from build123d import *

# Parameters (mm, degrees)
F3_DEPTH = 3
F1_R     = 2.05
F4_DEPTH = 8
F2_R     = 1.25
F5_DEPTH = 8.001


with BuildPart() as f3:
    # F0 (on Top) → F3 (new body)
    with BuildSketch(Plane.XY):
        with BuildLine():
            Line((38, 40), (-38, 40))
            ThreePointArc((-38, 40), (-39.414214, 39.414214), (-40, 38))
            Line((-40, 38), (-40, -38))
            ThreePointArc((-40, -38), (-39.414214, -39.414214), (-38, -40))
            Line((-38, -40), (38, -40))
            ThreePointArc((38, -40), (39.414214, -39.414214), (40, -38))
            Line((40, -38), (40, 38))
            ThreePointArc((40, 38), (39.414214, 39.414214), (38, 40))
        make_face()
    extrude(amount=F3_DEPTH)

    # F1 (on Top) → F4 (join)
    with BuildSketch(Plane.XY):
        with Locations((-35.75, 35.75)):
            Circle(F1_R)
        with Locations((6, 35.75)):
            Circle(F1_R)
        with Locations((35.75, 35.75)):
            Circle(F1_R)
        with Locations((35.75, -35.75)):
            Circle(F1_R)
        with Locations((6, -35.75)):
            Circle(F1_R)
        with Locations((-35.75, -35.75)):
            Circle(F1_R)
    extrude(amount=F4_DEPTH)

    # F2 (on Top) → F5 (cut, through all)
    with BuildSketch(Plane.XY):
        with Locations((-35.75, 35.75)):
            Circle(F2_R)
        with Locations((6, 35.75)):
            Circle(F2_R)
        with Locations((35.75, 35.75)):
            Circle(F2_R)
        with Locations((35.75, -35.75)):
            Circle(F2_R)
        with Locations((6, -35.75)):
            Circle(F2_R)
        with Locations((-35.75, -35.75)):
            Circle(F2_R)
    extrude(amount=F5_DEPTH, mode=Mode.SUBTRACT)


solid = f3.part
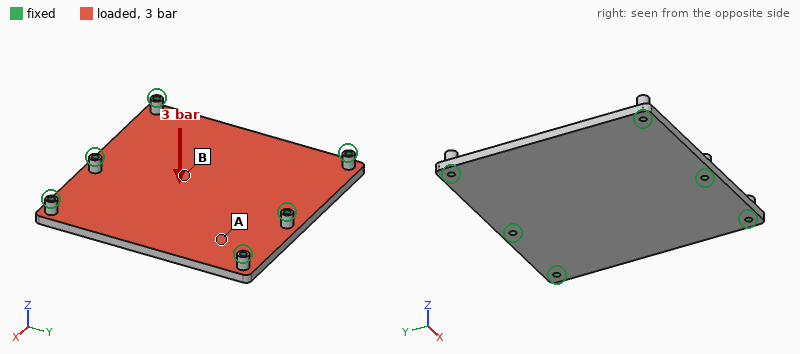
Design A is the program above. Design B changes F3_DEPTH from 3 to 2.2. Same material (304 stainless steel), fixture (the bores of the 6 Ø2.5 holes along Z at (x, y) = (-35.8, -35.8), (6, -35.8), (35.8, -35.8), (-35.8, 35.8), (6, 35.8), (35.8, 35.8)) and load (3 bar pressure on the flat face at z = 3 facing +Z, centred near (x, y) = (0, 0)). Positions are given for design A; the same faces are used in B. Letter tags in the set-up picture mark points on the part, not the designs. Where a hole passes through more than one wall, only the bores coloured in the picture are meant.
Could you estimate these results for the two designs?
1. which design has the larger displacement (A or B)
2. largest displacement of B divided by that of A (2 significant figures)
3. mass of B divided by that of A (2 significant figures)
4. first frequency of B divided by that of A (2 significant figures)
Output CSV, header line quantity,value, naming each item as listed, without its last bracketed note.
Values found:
quantity,value
which design has the larger displacement,B
largest displacement of B divided by that of A,2.4
mass of B divided by that of A,0.74
first frequency of B divided by that of A,0.75
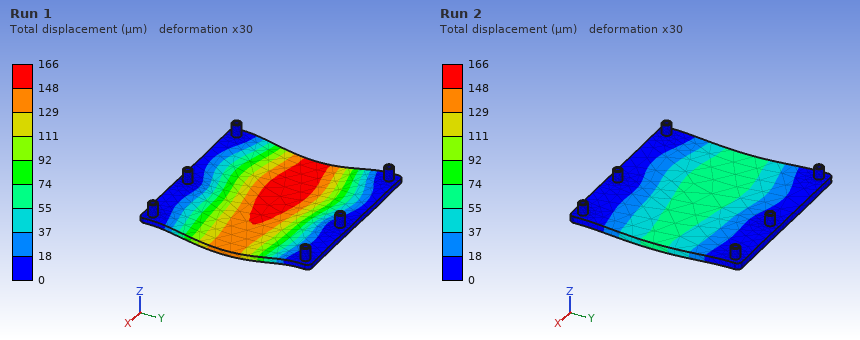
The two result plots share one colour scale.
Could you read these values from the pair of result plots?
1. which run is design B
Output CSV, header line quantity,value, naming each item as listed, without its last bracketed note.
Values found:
quantity,value
which run is design B,Run 1
